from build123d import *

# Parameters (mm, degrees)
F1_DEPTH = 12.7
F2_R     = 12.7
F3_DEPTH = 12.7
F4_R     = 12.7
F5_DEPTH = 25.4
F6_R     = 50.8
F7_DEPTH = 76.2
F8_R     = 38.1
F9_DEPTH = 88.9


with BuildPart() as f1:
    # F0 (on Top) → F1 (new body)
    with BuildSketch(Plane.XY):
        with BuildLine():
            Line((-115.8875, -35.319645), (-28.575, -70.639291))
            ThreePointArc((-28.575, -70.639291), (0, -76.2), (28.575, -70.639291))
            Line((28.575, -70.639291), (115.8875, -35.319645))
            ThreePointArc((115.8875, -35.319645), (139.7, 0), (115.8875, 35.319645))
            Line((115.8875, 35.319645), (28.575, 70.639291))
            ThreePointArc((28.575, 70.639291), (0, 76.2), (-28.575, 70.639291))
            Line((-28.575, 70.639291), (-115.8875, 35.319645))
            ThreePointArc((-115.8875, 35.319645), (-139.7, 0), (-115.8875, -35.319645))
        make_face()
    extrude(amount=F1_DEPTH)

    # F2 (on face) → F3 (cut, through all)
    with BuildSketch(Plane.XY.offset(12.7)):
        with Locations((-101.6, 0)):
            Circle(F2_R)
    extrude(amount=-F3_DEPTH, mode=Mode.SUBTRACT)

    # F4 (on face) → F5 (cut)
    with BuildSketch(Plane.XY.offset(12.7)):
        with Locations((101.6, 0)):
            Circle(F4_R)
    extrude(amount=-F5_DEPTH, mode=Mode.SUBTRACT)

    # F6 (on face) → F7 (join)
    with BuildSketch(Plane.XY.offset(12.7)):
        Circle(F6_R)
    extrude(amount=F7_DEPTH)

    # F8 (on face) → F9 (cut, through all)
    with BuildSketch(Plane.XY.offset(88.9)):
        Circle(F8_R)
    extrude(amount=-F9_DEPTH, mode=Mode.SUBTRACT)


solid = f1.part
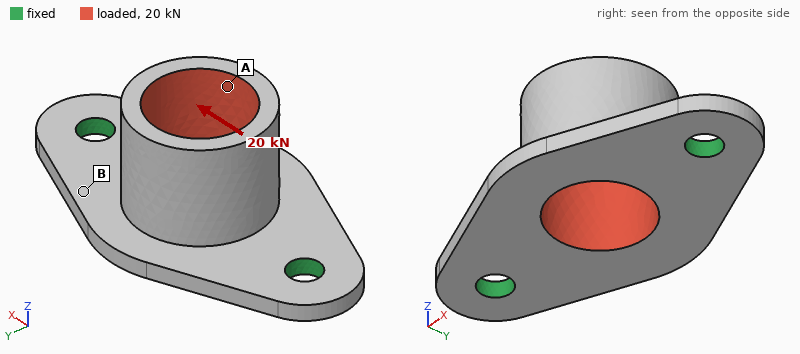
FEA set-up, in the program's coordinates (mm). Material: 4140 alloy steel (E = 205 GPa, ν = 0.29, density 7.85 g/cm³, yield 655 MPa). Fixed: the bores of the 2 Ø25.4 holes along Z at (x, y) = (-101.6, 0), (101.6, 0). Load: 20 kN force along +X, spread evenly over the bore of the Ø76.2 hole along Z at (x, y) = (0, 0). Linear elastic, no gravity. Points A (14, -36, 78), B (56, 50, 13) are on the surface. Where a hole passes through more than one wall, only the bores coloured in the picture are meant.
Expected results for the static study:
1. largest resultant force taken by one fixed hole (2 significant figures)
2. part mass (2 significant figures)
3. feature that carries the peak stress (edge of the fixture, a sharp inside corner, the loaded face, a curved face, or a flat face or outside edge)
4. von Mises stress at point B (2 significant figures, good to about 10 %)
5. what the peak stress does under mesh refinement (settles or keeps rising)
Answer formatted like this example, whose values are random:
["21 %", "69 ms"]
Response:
["11 kN", "4.5 kg", "edge of the fixture", "23 MPa", "keeps rising"]
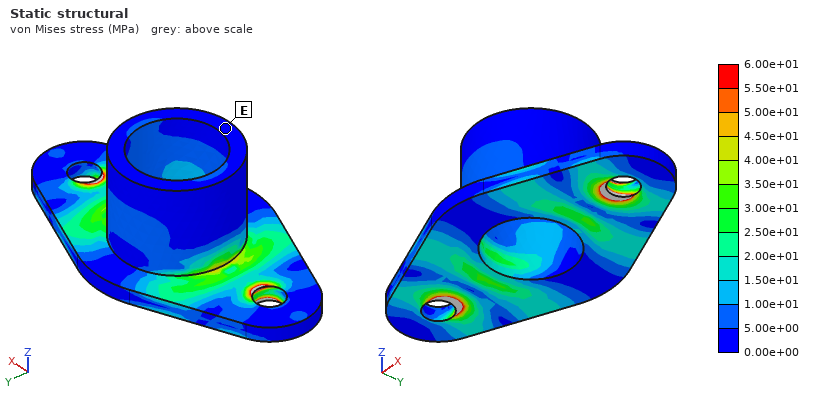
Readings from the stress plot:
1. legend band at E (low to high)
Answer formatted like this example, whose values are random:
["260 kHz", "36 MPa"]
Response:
["0.00e+00 to 5.00e+00 MPa"]
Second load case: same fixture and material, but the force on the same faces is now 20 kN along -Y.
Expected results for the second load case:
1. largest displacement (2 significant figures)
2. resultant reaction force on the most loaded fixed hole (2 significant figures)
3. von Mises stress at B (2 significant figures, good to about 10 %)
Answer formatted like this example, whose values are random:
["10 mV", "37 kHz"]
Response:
["0.31 mm", "10 kN", "45 MPa"]
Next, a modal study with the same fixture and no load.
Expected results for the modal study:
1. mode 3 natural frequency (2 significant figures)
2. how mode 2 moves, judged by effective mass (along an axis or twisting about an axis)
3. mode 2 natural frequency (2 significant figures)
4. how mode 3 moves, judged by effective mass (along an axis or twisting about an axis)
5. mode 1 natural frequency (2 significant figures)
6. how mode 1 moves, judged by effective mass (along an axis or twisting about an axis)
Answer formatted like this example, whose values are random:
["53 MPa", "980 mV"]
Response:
["2200 Hz", "along Z", "1500 Hz", "along X", "790 Hz", "along Y"]
